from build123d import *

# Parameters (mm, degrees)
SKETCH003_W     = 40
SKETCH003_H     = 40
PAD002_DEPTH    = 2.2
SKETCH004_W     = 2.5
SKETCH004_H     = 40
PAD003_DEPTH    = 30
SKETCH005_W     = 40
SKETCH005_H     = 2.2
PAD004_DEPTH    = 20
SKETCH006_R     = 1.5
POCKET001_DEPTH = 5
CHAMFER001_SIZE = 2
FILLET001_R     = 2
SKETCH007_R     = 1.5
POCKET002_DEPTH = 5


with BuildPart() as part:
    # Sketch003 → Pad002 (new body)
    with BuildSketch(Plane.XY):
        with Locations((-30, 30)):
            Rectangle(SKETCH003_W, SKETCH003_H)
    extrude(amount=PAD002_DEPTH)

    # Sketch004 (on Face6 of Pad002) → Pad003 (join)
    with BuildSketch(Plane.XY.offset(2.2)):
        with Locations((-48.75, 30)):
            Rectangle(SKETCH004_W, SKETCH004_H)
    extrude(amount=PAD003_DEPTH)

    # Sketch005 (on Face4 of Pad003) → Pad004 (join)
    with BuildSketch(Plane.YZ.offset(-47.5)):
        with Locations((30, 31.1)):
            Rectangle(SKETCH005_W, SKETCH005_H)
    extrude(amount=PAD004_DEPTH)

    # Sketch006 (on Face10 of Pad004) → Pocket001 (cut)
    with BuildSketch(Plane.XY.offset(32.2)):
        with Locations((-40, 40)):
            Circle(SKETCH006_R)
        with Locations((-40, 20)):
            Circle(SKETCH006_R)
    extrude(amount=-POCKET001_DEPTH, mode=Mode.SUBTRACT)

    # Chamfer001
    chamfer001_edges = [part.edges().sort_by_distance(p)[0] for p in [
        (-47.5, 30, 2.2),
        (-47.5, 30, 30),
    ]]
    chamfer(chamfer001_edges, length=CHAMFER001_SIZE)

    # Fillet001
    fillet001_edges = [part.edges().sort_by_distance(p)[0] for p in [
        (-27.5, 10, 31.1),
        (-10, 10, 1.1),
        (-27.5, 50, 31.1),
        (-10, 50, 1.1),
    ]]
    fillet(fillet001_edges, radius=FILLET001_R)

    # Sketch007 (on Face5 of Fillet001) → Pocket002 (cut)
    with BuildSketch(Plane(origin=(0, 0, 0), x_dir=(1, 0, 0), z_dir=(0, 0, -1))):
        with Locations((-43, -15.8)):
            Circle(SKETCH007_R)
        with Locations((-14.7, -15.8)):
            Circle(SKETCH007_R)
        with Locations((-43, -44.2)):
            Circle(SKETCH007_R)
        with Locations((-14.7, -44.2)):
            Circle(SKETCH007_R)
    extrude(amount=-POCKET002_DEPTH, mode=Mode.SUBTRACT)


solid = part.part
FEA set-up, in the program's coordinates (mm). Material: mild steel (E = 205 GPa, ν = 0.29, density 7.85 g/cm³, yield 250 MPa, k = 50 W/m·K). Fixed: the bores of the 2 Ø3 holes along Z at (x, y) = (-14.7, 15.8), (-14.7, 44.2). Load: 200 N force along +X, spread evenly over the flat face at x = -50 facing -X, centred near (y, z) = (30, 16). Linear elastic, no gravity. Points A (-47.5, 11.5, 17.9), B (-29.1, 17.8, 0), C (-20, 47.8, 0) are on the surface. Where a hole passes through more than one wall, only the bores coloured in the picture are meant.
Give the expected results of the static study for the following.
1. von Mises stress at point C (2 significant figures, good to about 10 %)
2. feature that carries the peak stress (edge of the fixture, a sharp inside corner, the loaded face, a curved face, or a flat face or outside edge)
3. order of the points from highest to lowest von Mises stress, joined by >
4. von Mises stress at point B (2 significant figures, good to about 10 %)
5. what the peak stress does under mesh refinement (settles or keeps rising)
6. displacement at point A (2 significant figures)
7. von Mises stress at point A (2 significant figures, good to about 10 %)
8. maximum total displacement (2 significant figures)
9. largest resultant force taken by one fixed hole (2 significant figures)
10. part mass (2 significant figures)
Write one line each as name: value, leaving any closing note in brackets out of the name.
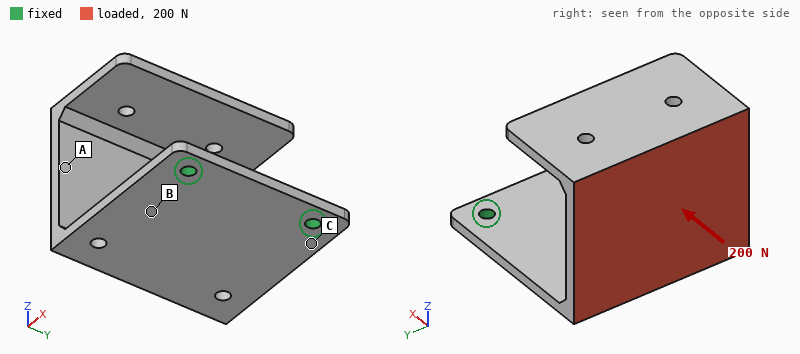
von Mises stress at point C: 110 MPa
feature that carries the peak stress: edge of the fixture
order of the points from highest to lowest von Mises stress, joined by >: C > B > A
von Mises stress at point B: 85 MPa
what the peak stress does under mesh refinement: keeps rising
displacement at point A: 0.34 mm
von Mises stress at point A: 15 MPa
maximum total displacement: 0.54 mm
largest resultant force taken by one fixed hole: 100 N
part mass: 65 g
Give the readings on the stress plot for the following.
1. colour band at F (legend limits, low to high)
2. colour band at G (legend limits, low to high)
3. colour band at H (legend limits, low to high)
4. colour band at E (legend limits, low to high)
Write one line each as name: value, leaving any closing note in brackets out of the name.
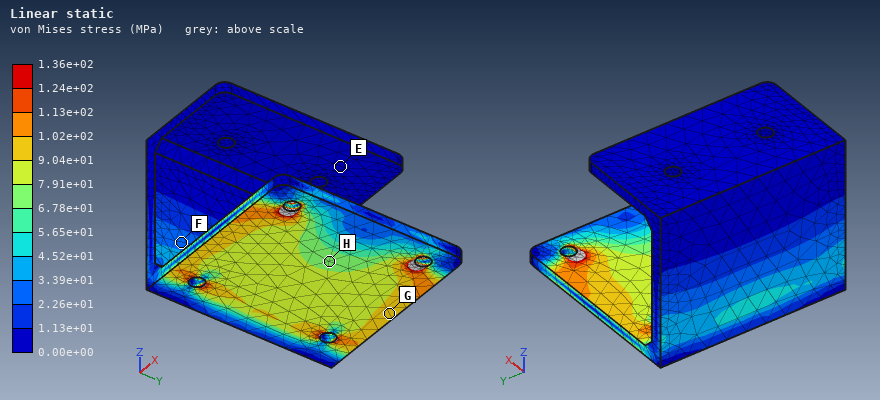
colour band at F: 2.26e+01 to 3.39e+01 MPa
colour band at G: 9.04e+01 to 1.02e+02 MPa
colour band at H: 6.78e+01 to 7.91e+01 MPa
colour band at E: 0.00e+00 to 1.13e+01 MPa
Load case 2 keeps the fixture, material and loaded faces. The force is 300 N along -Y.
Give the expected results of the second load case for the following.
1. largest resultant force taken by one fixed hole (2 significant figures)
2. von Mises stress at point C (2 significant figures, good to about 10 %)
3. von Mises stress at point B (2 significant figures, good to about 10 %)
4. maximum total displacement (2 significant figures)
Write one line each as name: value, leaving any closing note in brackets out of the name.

largest resultant force taken by one fixed hole: 410 N
von Mises stress at point C: 110 MPa
von Mises stress at point B: 80 MPa
maximum total displacement: 0.29 mm
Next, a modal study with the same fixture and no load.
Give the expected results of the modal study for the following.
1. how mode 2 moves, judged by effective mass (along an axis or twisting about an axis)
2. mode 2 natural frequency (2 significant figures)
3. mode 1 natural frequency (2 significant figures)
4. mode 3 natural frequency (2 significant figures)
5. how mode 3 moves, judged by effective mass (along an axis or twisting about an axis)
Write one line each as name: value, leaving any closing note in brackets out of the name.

how mode 2 moves, judged by effective mass: along Y
mode 2 natural frequency: 720 Hz
mode 1 natural frequency: 400 Hz
mode 3 natural frequency: 1000 Hz
how mode 3 moves, judged by effective mass: along Z
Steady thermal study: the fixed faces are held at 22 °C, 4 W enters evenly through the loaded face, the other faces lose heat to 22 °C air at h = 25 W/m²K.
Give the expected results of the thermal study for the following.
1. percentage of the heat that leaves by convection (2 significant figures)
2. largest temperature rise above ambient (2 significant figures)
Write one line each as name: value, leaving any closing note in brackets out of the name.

percentage of the heat that leaves by convection: 55 %
largest temperature rise above ambient: 22 K
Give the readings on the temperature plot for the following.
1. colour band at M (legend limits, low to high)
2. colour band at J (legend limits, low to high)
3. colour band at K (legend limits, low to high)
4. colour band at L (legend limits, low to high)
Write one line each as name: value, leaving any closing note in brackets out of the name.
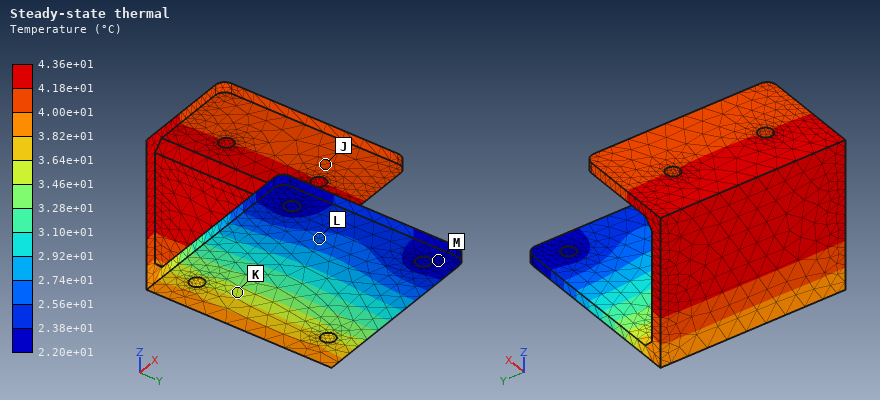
colour band at M: 2.20e+01 to 2.38e+01 °C
colour band at J: 4.00e+01 to 4.18e+01 °C
colour band at K: 3.46e+01 to 3.64e+01 °C
colour band at L: 2.56e+01 to 2.74e+01 °C
